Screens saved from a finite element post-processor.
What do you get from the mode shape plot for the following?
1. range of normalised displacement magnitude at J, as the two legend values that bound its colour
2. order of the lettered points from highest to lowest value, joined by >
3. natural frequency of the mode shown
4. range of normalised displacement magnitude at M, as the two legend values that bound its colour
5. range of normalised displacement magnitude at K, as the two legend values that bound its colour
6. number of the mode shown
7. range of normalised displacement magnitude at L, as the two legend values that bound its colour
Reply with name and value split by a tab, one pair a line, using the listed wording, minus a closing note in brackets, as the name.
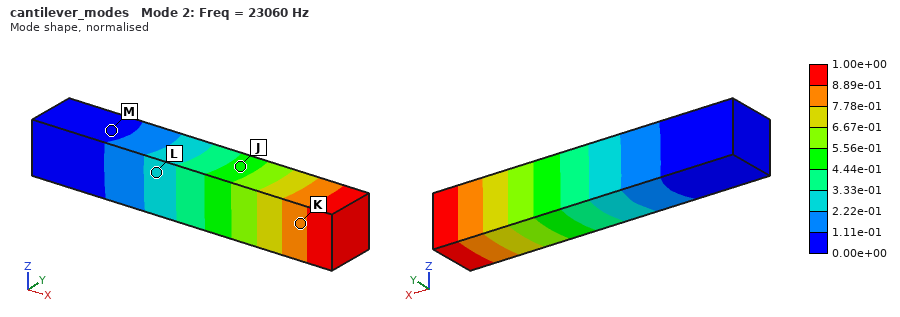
range of normalised displacement magnitude at J, as the two legend values that bound its colour	4.44e-01 to 5.56e-01
order of the lettered points from highest to lowest value, joined by >	K > J > L > M
natural frequency of the mode shown	23060 Hz
range of normalised displacement magnitude at M, as the two legend values that bound its colour	0.00e+00 to 1.11e-01
range of normalised displacement magnitude at K, as the two legend values that bound its colour	7.78e-01 to 8.89e-01
number of the mode shown	2
range of normalised displacement magnitude at L, as the two legend values that bound its colour	2.22e-01 to 3.33e-01
